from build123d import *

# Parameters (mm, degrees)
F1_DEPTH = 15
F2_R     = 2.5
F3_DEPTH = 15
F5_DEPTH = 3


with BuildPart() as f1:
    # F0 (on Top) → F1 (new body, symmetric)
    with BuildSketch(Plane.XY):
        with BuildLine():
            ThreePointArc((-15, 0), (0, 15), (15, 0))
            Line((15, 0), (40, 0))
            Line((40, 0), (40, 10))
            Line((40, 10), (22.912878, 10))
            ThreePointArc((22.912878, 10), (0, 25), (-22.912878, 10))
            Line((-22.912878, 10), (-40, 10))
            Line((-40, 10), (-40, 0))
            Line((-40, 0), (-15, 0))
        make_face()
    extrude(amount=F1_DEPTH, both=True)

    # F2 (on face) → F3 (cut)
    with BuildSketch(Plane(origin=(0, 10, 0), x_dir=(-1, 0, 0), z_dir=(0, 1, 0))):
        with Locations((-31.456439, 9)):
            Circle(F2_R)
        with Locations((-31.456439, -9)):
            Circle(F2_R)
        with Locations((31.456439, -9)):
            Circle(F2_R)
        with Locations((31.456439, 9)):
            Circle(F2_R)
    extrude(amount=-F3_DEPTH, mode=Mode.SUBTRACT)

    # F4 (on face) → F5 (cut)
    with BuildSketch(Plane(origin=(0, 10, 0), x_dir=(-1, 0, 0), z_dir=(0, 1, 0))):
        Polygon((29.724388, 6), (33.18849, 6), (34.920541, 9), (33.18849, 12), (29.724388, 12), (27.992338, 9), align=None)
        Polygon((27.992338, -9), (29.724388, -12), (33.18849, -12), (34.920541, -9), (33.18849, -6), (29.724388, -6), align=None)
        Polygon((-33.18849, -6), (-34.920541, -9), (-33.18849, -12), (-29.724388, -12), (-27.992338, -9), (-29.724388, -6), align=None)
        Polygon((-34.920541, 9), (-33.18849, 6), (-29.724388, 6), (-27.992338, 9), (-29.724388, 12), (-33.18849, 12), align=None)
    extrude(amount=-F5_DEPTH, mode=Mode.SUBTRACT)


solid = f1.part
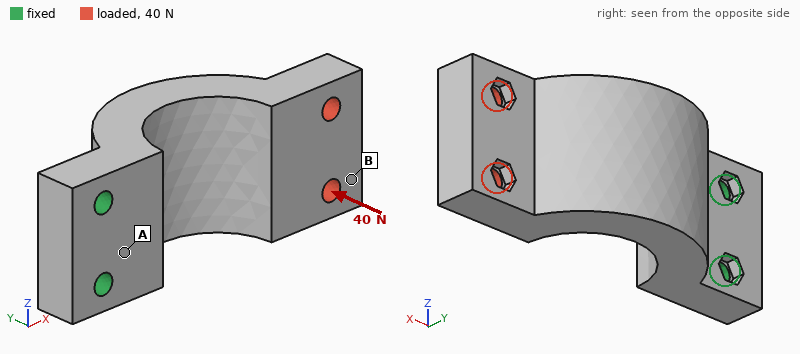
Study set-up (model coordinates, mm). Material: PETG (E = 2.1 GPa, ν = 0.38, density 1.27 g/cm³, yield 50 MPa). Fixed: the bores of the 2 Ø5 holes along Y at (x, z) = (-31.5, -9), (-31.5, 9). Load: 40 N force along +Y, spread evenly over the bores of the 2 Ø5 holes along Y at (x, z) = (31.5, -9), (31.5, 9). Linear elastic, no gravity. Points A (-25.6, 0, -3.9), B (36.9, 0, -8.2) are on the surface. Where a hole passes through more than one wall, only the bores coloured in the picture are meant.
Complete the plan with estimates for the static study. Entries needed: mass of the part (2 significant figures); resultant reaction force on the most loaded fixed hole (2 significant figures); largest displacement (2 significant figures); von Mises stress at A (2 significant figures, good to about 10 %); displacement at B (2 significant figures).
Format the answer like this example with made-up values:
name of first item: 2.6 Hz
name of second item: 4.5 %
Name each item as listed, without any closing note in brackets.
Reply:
mass of the part: 35 g
resultant reaction force on the most loaded fixed hole: 20 N
largest displacement: 1.00 mm
von Mises stress at A: 3.9 MPa
displacement at B: 0.94 mm
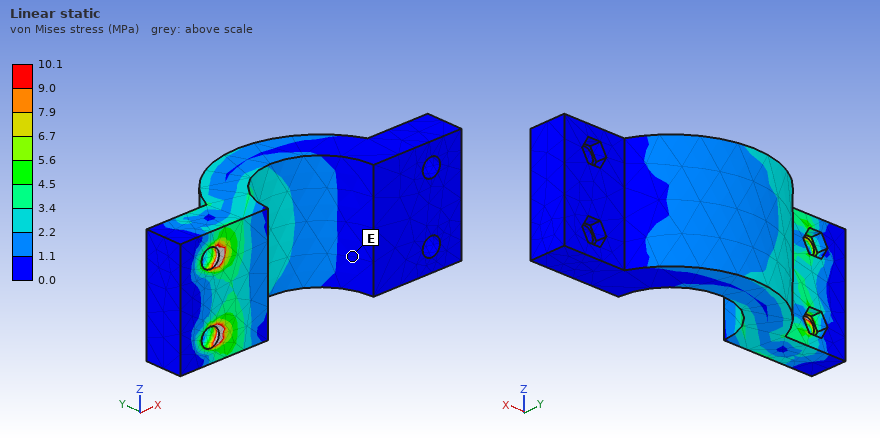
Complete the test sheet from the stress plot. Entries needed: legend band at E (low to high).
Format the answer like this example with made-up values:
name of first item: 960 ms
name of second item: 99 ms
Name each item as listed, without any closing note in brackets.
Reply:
legend band at E: 0.0 to 1.1 MPa
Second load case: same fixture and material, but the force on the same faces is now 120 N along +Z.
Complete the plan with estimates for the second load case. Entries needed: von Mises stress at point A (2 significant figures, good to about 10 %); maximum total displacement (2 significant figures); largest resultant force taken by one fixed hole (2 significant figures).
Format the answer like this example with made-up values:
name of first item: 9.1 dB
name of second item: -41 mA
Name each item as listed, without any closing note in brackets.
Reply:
von Mises stress at point A: 4.6 MPa
maximum total displacement: 0.97 mm
largest resultant force taken by one fixed hole: 370 N
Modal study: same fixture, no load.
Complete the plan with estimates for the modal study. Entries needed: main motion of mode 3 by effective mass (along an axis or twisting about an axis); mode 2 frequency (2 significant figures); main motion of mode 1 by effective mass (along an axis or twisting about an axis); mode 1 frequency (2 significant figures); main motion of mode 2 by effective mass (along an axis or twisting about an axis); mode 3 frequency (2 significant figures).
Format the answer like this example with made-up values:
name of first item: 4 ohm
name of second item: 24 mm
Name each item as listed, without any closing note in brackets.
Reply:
main motion of mode 3 by effective mass: along X
mode 2 frequency: 630 Hz
main motion of mode 1 by effective mass: along Y
mode 1 frequency: 340 Hz
main motion of mode 2 by effective mass: along Z
mode 3 frequency: 1200 Hz
